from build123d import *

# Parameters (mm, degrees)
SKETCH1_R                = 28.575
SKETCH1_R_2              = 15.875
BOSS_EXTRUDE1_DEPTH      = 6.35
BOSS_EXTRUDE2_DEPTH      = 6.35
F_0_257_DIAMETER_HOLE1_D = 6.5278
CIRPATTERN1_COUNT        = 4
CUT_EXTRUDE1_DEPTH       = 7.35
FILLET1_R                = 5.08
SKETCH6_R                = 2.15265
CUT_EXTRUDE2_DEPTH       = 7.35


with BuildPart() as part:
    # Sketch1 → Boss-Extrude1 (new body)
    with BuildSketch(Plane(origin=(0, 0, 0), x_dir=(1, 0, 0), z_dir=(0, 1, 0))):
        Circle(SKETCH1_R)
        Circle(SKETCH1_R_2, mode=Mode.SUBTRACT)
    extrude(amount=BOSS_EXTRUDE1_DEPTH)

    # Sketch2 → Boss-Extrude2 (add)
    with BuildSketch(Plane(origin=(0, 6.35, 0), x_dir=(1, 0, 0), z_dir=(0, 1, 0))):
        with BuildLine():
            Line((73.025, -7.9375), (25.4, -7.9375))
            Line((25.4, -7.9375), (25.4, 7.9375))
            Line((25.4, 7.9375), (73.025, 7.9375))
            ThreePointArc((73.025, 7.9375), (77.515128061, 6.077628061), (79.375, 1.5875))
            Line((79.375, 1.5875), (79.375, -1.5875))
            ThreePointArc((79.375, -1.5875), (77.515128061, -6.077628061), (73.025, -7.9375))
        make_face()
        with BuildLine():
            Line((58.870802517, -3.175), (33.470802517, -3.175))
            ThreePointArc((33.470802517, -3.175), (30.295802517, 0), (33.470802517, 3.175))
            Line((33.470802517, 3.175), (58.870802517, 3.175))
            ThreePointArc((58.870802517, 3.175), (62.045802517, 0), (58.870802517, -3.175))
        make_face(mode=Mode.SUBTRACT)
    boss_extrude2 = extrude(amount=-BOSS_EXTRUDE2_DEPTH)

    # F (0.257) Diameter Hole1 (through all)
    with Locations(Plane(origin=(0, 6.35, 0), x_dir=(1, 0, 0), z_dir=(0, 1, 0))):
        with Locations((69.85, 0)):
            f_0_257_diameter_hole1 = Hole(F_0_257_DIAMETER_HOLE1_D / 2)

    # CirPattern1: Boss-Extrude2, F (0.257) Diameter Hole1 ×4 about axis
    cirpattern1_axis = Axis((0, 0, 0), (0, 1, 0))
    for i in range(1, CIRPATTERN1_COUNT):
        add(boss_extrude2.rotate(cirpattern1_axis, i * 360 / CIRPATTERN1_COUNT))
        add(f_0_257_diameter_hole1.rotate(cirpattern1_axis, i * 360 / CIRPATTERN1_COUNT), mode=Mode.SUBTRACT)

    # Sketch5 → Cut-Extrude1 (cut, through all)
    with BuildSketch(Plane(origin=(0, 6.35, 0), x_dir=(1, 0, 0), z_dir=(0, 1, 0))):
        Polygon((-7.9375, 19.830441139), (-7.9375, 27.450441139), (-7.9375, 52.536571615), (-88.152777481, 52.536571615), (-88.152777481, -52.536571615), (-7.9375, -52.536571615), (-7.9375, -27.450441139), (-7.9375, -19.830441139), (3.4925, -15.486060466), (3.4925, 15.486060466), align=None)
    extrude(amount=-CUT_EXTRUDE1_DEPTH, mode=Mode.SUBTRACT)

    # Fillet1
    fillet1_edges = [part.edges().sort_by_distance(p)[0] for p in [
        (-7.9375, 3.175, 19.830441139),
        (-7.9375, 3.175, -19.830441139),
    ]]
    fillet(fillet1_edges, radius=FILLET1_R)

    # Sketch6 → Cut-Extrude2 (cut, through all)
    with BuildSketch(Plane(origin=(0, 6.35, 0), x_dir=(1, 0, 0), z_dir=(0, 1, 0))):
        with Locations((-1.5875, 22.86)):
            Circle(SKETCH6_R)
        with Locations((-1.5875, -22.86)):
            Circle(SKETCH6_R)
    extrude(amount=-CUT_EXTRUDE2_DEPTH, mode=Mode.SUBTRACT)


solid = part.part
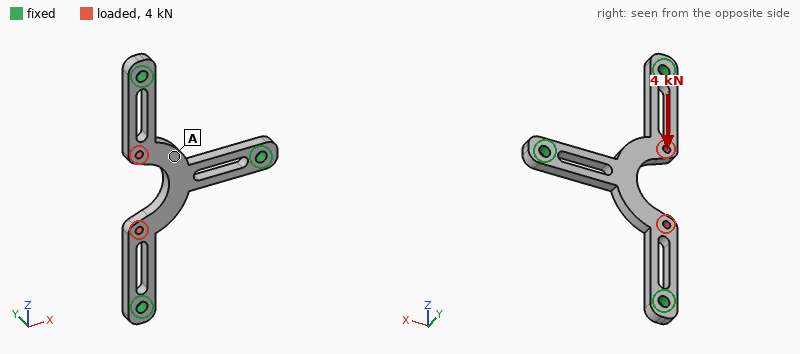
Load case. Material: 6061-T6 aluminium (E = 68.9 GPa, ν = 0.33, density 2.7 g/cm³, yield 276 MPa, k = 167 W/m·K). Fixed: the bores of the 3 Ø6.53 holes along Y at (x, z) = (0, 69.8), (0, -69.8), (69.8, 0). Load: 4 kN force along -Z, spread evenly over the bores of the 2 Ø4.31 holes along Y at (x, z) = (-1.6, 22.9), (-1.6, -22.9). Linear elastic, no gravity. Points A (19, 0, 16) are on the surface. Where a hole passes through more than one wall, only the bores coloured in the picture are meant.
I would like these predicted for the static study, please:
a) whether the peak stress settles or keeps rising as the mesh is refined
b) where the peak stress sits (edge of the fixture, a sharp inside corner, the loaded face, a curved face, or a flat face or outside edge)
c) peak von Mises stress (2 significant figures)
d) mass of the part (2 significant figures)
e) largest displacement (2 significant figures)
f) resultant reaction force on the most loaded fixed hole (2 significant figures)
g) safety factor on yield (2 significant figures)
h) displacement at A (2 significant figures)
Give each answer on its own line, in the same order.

settles
a curved face
63 MPa
47 g
26 µm
2.0 kN
4.4
13 µm
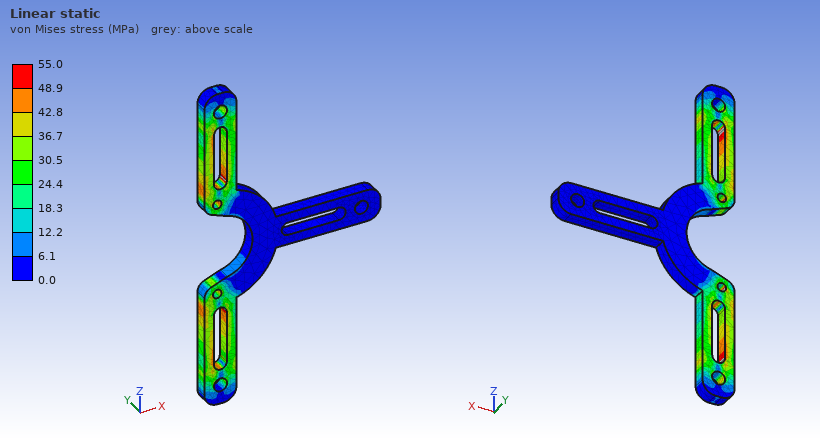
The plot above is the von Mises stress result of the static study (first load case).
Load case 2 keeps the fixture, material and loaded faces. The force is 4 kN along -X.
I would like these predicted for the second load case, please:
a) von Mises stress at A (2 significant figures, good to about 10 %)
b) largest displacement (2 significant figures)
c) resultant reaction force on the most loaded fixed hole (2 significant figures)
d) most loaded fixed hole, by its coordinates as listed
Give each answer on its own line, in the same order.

28 MPa
69 µm
3.7 kN
(69.8, 0)
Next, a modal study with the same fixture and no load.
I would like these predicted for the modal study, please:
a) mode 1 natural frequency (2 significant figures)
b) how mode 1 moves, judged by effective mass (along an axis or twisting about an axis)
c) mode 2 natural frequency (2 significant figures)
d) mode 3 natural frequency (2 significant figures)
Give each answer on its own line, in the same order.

1900 Hz
along Y
3800 Hz
5100 Hz
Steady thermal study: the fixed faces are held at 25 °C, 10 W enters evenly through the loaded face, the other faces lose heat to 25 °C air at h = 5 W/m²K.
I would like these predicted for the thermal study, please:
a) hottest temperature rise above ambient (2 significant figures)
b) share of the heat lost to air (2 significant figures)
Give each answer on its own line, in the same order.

15 K
3.4 %
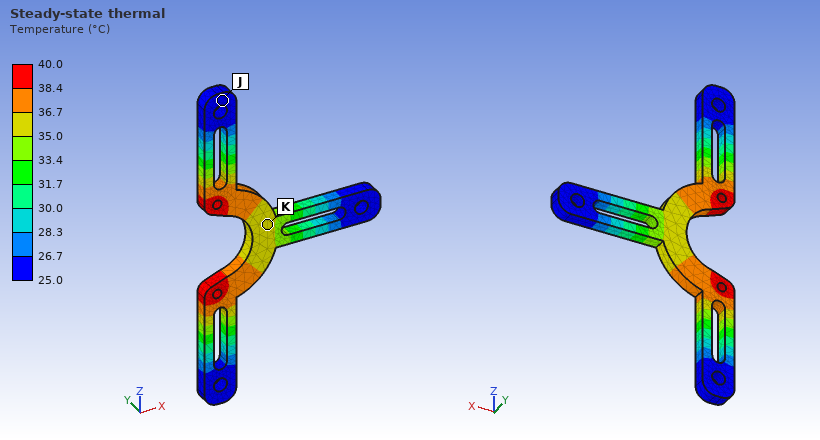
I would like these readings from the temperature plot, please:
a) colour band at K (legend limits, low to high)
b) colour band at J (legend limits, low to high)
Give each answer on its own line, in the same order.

35.0 to 36.7 °C
25.0 to 26.7 °C
